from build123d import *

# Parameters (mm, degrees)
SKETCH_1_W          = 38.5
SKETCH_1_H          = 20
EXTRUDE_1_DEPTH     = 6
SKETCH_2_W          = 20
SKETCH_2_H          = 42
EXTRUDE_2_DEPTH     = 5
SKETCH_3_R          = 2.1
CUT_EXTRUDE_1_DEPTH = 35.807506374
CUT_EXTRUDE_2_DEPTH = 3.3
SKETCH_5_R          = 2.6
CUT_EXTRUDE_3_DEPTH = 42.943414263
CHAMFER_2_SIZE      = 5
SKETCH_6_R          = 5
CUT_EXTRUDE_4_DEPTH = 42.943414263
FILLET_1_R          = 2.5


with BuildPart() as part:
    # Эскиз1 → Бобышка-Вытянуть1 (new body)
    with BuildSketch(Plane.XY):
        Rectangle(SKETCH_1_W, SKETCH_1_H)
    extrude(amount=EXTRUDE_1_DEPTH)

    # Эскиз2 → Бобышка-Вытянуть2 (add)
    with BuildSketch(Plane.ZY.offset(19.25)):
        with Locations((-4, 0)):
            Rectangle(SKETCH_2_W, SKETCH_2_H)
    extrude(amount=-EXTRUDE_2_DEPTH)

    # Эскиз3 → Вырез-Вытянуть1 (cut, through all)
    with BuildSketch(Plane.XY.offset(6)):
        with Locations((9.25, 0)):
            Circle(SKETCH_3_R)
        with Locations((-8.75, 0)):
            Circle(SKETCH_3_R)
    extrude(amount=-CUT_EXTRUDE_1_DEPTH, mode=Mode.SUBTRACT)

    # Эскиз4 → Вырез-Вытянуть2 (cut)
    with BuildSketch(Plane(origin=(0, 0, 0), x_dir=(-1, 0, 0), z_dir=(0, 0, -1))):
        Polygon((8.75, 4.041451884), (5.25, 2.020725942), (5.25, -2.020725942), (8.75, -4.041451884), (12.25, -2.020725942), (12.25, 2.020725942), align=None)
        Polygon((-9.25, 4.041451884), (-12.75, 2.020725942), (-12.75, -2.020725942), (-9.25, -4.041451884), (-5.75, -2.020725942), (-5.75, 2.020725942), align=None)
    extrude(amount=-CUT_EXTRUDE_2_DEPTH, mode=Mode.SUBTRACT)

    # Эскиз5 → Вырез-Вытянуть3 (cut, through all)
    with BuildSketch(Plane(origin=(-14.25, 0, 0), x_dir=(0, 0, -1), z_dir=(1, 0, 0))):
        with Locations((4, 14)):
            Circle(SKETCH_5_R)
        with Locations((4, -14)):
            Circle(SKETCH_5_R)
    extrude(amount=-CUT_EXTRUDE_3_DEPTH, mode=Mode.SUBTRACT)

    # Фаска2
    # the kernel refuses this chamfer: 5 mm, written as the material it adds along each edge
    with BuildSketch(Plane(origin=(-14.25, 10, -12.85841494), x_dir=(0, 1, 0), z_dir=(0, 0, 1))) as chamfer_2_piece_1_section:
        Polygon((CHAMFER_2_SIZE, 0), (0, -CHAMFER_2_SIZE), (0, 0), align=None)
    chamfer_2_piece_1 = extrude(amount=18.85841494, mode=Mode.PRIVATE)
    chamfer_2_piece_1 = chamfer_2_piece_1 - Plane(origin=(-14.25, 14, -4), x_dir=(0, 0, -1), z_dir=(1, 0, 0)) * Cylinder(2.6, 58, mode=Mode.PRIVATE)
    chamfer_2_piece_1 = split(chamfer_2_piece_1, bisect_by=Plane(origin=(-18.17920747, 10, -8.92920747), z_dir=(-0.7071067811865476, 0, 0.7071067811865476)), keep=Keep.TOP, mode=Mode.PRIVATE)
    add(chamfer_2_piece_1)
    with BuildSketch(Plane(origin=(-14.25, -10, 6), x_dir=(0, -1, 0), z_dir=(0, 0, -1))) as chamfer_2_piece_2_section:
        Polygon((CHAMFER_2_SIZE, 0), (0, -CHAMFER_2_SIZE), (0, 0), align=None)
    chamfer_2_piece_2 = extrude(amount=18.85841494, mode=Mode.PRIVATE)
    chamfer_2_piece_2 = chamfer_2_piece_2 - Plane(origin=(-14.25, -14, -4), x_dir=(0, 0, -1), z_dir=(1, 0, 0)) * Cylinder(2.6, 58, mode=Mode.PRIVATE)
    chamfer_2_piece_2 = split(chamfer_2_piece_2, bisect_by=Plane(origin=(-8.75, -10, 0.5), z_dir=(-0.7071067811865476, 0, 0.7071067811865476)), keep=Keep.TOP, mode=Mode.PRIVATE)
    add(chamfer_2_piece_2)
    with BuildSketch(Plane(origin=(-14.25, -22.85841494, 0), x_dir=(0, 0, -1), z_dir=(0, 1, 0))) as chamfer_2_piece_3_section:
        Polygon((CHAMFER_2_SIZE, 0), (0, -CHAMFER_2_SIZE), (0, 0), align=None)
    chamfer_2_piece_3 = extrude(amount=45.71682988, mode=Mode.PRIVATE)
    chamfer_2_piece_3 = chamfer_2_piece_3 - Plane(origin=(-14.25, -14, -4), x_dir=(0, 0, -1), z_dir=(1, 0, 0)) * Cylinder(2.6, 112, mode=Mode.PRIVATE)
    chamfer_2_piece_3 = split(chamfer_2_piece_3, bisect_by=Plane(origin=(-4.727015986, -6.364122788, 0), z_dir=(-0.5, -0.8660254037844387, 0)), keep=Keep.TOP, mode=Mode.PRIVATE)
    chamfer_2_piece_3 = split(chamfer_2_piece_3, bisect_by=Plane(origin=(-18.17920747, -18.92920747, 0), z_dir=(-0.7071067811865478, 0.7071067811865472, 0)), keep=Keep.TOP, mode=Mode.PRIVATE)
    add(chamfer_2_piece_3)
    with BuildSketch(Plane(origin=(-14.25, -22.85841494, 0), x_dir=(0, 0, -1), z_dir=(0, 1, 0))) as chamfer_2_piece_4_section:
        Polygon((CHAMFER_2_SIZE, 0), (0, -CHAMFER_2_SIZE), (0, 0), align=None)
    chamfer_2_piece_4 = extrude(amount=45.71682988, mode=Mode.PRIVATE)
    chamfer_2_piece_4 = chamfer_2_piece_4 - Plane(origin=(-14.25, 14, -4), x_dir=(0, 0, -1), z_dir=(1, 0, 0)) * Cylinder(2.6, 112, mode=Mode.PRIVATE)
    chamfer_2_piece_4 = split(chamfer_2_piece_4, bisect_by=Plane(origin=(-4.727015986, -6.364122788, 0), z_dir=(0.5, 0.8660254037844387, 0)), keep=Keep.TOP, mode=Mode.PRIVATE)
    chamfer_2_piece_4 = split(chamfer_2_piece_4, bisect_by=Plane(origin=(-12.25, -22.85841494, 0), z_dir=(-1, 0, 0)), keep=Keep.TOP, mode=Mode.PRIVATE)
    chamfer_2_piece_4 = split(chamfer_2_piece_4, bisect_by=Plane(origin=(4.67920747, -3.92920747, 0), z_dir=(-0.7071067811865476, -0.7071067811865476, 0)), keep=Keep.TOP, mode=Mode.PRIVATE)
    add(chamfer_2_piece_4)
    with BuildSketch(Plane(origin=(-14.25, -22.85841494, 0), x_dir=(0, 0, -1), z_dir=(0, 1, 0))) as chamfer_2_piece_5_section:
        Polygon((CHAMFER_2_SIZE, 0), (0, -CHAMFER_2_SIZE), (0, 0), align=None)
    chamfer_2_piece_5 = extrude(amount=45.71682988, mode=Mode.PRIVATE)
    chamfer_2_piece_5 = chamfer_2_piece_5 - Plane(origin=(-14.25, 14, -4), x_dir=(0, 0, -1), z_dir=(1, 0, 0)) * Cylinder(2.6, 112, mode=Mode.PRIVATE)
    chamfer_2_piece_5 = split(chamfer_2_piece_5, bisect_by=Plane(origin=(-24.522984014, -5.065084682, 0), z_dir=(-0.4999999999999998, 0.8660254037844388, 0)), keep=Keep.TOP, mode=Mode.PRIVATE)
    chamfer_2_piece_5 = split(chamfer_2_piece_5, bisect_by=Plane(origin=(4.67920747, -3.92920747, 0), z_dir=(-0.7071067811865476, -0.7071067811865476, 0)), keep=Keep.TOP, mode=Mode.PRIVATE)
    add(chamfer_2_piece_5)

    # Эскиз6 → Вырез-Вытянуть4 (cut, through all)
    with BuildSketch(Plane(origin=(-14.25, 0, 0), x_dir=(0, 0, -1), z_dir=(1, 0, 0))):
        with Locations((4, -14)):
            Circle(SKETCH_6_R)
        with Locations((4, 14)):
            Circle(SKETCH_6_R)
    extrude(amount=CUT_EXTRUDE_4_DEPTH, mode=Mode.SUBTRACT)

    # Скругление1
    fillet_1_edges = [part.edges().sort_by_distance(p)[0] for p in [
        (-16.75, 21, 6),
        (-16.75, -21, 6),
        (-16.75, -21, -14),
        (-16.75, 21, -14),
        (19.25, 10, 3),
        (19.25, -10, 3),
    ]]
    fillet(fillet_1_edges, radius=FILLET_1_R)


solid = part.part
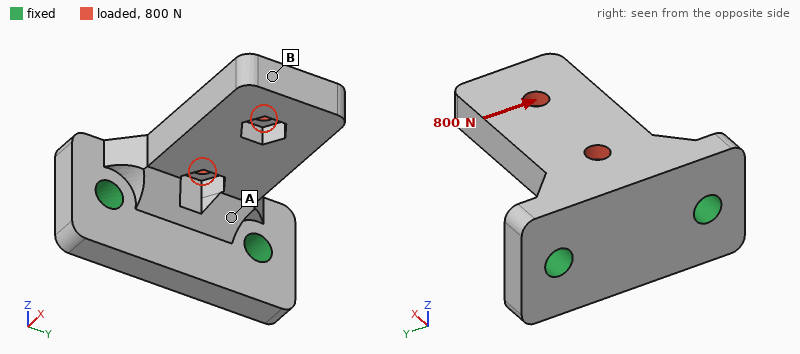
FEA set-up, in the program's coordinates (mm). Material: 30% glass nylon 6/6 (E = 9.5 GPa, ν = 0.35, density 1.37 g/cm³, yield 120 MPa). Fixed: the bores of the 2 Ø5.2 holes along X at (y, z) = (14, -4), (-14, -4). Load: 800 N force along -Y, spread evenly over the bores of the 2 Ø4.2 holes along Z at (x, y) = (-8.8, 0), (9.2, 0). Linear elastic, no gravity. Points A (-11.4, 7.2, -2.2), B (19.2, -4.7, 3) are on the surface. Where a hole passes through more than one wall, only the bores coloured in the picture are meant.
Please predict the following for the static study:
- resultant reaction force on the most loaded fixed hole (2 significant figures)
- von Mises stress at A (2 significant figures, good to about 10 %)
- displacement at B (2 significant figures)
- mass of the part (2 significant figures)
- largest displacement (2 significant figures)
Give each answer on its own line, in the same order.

700 N
15 MPa
0.18 mm
11 g
0.18 mm
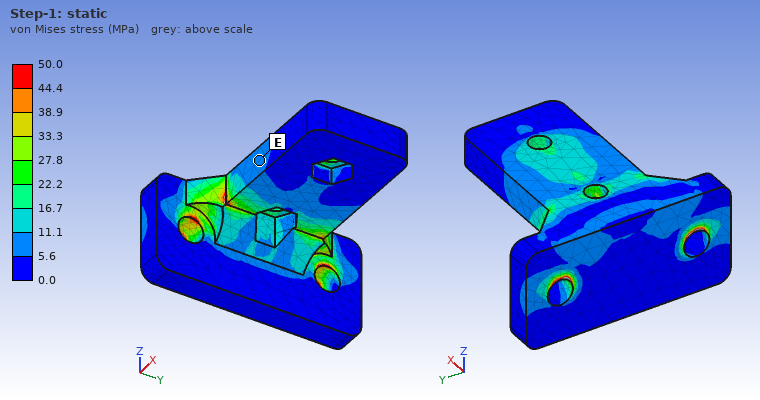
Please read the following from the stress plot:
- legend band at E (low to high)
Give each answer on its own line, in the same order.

5.6 to 11.1 MPa
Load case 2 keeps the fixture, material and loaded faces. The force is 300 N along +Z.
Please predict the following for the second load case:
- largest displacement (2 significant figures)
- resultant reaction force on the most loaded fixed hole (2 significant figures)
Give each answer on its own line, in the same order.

0.57 mm
150 N
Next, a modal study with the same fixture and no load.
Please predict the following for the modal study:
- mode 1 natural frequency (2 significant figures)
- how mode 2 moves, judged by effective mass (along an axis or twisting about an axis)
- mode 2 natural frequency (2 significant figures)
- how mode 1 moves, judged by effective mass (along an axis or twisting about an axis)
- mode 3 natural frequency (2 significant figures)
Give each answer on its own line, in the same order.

1800 Hz
along Y
4900 Hz
along Z
6900 Hz
